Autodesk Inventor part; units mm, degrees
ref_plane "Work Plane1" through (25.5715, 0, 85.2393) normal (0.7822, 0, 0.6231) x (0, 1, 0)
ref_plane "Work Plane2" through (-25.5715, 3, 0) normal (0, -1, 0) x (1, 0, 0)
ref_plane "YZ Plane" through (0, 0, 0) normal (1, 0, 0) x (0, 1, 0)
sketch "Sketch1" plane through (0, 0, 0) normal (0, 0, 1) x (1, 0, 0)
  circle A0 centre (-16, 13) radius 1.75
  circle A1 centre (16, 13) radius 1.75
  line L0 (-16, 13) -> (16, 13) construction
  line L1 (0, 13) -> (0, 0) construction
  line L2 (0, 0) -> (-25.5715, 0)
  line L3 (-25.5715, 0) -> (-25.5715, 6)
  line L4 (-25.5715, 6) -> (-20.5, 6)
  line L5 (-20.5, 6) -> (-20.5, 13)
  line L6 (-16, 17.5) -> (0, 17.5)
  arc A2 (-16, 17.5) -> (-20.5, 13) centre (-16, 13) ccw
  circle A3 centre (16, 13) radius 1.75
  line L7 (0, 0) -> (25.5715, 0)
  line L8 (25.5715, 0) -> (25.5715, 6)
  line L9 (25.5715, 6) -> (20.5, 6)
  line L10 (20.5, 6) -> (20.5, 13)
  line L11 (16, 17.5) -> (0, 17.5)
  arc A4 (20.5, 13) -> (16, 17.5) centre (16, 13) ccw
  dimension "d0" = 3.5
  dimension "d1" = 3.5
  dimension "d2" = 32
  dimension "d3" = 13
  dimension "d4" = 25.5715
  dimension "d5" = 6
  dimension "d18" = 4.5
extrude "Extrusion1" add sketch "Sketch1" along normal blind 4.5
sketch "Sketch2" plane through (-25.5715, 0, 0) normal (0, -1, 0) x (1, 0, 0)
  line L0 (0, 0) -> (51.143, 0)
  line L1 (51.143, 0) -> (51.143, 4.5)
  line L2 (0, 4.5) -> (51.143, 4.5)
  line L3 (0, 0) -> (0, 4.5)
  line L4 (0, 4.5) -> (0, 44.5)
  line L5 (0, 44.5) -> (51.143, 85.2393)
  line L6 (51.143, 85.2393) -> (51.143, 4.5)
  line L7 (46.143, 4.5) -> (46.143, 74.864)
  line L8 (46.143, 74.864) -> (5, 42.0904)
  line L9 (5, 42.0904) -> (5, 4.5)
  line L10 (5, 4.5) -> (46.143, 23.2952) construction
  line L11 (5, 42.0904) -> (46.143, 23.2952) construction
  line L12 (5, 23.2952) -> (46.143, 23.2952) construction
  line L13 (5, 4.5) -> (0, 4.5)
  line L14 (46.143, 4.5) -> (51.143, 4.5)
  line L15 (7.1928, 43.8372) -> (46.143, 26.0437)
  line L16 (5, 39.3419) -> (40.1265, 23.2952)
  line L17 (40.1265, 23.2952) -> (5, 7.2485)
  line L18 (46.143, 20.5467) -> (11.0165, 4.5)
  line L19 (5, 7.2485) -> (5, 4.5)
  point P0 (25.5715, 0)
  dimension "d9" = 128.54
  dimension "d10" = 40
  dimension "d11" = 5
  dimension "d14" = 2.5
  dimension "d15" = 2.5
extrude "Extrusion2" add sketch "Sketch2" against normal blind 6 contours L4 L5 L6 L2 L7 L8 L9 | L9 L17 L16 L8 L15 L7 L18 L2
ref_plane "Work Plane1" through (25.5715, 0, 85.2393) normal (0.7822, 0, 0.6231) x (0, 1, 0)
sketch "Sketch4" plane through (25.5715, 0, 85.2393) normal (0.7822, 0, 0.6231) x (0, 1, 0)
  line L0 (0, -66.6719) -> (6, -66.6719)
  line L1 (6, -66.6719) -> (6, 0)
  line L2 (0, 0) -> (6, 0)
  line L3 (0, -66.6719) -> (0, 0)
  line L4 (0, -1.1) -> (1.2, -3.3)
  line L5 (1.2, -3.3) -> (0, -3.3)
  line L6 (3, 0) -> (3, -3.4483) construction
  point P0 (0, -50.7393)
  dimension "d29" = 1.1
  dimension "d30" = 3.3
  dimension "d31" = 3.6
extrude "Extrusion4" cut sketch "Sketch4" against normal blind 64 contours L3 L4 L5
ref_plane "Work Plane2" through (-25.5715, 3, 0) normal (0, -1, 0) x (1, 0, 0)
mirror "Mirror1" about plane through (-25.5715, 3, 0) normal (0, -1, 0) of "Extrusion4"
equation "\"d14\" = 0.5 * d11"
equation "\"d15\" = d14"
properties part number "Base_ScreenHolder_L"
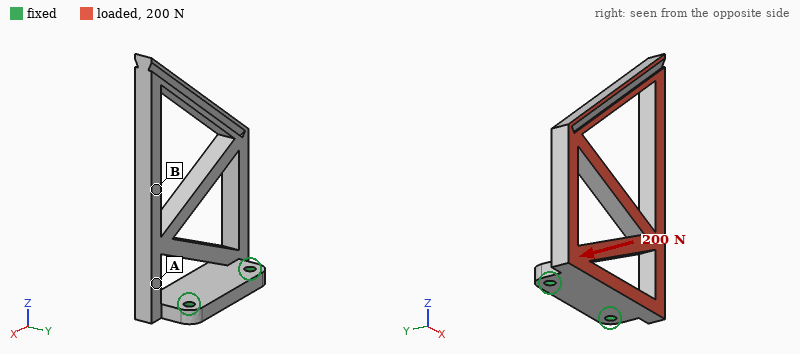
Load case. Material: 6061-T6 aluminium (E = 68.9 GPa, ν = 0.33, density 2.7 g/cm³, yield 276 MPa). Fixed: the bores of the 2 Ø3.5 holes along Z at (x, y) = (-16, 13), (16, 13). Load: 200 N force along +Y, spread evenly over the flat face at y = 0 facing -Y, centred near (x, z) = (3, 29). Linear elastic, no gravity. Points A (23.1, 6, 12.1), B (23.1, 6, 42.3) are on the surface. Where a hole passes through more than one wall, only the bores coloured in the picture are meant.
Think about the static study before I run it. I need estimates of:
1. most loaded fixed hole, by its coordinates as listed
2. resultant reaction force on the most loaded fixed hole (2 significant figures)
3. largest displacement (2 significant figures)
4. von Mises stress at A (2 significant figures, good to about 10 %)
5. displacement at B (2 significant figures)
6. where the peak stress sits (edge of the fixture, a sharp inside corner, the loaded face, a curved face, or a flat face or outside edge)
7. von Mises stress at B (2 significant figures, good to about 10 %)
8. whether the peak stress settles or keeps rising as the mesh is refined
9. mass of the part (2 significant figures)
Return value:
(16, 13)
110 N
1.0 mm
53 MPa
0.41 mm
a sharp inside corner
18 MPa
keeps rising
30 g
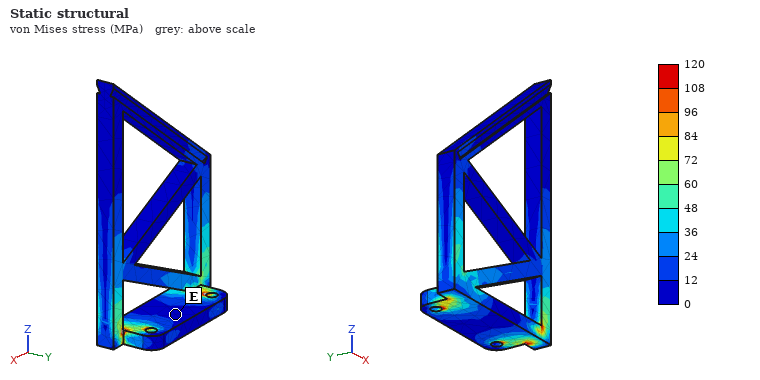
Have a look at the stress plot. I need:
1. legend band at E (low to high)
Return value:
0 to 12 MPa
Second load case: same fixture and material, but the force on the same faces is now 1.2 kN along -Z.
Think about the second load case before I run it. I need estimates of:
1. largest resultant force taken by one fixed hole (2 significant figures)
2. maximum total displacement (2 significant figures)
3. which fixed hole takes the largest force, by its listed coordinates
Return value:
680 N
1.1 mm
(16, 13)
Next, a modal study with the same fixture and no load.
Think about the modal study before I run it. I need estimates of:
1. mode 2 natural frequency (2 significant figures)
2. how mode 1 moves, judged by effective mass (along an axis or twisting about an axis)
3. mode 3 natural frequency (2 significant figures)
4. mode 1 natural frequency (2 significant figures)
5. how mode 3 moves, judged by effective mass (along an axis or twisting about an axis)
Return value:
1900 Hz
along Y
2400 Hz
580 Hz
along X
